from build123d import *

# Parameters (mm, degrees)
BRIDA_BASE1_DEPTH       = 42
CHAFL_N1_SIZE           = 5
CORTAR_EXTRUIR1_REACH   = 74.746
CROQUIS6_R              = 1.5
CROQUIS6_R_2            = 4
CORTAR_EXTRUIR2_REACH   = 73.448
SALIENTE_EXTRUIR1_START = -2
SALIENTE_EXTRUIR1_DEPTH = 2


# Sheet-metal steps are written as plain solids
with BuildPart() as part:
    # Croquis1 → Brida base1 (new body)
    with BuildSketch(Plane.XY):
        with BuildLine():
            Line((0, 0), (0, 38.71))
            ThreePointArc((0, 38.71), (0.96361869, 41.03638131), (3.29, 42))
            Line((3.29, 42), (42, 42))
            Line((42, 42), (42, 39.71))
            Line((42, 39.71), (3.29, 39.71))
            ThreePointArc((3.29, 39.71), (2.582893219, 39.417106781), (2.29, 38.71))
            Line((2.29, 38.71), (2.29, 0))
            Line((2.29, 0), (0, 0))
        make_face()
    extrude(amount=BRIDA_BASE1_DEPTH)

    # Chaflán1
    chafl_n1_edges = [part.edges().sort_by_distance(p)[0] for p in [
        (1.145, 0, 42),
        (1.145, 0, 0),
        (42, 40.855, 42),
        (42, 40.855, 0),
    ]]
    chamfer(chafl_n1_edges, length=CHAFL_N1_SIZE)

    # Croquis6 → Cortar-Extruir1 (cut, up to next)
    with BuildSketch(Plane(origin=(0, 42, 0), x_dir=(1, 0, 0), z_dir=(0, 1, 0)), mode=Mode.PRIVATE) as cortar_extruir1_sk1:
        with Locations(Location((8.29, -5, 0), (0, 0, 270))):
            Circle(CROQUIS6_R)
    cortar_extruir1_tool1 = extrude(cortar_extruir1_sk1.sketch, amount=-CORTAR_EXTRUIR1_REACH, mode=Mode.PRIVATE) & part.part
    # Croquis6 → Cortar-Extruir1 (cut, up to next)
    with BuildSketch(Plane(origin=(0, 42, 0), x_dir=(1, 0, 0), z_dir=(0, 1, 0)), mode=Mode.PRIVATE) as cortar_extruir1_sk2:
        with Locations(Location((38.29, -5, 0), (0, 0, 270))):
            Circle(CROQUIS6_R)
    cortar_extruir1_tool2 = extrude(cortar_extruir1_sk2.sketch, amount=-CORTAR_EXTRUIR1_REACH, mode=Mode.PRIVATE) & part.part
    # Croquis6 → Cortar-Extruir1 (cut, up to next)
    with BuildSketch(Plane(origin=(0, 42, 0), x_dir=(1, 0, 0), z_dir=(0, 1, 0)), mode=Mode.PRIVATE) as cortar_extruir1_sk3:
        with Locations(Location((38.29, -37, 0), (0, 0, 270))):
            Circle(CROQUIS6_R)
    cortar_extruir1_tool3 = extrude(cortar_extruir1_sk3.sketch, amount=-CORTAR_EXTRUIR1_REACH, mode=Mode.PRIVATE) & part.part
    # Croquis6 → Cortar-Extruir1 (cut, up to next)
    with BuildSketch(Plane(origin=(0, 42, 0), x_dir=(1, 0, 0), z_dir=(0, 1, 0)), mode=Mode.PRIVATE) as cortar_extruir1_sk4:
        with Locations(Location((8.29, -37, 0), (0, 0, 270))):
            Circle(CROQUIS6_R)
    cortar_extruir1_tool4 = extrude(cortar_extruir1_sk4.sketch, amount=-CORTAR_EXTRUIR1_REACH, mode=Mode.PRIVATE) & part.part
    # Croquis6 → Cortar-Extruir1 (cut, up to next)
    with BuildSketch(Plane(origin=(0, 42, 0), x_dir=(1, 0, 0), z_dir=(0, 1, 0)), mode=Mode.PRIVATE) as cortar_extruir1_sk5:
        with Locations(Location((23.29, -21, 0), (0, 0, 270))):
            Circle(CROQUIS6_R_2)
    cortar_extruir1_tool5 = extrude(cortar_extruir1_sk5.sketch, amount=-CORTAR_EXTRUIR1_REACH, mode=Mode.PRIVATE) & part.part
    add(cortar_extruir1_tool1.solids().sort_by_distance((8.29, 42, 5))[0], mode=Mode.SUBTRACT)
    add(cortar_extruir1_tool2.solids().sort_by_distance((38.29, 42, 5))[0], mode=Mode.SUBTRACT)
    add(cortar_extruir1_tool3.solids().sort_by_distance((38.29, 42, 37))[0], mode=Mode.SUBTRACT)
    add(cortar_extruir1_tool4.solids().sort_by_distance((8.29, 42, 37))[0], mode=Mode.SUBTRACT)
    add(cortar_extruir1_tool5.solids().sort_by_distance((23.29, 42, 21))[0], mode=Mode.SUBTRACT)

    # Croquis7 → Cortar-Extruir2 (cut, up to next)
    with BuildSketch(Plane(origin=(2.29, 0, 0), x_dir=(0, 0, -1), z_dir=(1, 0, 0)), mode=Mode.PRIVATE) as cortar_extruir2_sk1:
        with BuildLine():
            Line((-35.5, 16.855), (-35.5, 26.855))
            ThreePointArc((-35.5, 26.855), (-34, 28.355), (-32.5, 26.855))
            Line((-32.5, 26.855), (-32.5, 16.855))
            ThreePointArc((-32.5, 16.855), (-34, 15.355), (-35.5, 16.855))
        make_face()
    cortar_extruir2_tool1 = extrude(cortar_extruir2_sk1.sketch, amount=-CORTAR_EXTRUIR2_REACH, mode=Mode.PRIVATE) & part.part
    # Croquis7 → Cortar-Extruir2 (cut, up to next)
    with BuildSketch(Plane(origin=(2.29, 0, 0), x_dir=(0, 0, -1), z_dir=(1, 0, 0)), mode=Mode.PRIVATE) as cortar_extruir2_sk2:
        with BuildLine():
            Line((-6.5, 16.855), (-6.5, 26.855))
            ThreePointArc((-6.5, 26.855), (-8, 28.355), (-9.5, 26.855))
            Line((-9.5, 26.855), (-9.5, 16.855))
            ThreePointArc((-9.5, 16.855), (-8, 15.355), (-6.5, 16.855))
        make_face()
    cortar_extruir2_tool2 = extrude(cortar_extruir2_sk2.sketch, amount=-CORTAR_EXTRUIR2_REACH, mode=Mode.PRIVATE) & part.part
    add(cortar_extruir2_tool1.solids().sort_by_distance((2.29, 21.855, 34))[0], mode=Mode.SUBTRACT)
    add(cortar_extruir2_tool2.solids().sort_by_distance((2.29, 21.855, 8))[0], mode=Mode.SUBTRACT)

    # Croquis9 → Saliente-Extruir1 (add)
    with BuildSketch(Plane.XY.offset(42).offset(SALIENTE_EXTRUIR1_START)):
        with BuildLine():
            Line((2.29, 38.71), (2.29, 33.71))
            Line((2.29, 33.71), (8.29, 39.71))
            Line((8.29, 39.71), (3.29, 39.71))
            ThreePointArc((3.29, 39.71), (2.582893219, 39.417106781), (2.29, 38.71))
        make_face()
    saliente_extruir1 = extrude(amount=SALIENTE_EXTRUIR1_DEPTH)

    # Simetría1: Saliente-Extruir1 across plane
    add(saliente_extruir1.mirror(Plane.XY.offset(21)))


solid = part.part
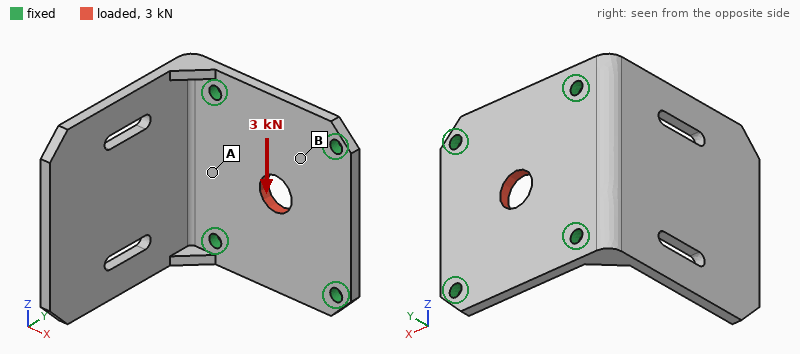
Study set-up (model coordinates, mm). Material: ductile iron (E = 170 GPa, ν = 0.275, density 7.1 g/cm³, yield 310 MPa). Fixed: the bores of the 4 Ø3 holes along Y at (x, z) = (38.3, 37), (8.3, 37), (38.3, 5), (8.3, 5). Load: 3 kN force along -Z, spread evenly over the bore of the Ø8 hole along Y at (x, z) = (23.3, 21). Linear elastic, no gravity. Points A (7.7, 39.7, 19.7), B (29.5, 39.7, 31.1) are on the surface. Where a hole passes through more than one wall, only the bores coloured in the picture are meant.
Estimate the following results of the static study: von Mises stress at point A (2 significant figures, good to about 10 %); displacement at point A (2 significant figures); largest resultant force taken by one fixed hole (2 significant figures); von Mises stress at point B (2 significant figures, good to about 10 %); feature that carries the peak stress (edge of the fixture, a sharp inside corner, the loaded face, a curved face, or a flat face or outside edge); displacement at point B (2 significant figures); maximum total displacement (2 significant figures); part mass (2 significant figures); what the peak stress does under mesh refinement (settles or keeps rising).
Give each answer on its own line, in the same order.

11 MPa
1.3 µm
840 N
33 MPa
edge of the fixture
3.0 µm
5.3 µm
52 g
keeps rising
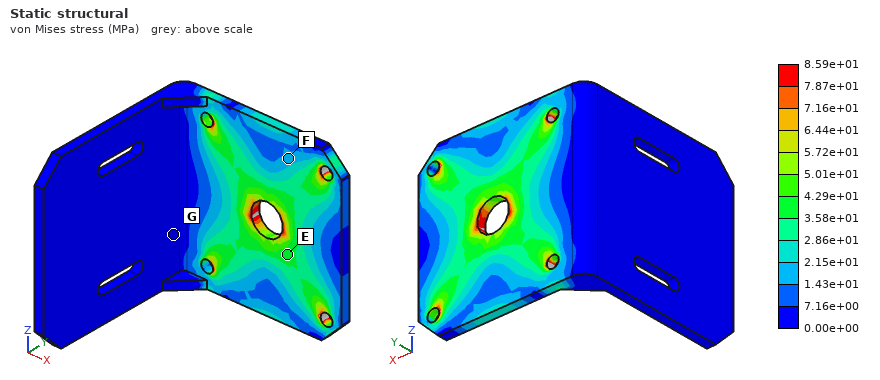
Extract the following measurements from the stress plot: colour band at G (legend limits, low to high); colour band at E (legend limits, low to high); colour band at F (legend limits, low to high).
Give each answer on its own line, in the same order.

0.00e+00 to 7.16e+00 MPa
3.58e+01 to 4.29e+01 MPa
1.43e+01 to 2.15e+01 MPa
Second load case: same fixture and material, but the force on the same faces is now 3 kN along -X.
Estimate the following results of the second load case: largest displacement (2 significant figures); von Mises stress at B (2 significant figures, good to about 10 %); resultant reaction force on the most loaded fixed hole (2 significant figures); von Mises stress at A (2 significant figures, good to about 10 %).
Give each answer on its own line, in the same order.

5.7 µm
33 MPa
860 N
13 MPa
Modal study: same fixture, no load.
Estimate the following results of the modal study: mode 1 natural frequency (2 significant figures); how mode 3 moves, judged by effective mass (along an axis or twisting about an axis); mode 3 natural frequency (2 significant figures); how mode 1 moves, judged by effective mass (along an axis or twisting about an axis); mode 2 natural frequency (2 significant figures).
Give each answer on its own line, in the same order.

970 Hz
along Z
4900 Hz
along X
2600 Hz
